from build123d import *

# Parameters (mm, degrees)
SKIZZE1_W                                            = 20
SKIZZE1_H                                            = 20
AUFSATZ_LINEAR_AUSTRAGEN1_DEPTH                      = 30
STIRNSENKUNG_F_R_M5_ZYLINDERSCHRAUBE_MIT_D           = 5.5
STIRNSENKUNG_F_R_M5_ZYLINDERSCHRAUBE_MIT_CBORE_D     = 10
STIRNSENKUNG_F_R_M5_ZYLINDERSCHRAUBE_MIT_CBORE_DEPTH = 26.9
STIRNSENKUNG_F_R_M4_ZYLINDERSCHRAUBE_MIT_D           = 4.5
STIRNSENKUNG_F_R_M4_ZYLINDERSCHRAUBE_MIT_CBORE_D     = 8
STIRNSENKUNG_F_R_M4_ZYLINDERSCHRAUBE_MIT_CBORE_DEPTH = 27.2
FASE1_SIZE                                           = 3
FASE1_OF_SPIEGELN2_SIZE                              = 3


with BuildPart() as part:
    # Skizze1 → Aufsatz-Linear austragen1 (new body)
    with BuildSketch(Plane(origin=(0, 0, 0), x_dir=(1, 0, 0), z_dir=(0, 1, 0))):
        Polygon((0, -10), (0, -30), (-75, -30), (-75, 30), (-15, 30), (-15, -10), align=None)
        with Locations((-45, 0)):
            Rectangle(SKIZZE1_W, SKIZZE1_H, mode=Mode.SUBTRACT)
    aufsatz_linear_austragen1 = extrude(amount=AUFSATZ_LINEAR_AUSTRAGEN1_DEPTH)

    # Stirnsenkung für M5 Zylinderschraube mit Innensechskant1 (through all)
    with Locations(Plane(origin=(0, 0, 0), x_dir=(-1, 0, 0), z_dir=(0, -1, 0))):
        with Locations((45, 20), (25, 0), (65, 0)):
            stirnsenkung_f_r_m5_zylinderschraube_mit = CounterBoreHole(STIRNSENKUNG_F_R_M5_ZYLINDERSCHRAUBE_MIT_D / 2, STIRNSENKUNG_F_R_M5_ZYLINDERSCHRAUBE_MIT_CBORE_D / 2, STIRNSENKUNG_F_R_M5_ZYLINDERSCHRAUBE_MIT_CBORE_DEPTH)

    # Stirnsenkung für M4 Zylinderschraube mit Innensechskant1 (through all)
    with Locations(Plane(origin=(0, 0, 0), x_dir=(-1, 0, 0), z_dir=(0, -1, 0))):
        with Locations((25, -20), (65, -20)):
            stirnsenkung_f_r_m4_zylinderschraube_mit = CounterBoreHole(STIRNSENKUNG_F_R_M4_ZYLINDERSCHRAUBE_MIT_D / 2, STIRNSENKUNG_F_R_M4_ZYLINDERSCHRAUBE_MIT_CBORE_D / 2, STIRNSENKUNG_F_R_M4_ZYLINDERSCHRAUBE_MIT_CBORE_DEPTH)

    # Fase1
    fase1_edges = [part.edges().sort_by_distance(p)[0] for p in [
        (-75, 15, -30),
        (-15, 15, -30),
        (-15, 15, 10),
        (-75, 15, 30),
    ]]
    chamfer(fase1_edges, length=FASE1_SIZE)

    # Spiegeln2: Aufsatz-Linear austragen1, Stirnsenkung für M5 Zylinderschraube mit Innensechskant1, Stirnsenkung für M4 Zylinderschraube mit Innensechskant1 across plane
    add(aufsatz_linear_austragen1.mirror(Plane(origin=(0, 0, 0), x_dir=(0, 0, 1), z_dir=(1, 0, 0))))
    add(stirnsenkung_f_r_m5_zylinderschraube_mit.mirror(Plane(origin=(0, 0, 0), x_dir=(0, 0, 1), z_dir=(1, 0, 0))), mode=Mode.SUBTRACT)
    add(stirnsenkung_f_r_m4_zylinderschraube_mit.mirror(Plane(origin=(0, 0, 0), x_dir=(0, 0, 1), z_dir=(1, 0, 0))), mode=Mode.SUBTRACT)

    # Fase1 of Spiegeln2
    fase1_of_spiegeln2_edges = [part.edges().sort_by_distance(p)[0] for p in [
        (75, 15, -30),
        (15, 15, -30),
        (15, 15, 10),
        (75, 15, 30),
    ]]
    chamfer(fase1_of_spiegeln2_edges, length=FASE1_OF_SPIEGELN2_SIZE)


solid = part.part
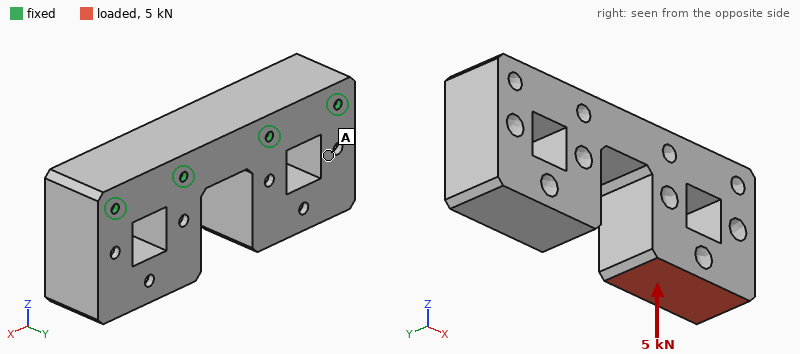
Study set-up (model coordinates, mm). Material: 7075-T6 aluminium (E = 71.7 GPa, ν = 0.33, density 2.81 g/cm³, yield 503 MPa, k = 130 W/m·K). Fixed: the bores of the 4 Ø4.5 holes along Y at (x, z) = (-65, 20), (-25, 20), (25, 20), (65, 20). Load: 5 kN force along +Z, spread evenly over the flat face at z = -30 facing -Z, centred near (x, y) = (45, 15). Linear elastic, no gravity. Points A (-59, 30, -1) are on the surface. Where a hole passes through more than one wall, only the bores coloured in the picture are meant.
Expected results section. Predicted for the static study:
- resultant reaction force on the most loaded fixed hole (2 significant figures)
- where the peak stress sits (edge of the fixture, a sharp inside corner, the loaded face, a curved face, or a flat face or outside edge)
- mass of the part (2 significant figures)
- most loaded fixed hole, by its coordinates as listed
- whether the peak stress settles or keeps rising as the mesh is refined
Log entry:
2.8 kN
edge of the fixture
540 g
(65, 20)
keeps rising
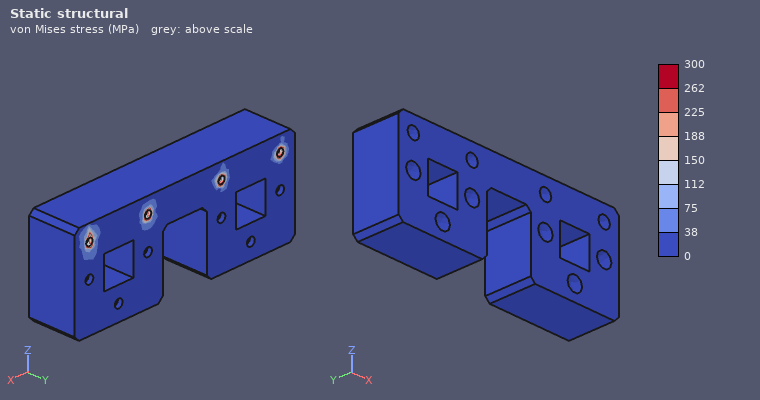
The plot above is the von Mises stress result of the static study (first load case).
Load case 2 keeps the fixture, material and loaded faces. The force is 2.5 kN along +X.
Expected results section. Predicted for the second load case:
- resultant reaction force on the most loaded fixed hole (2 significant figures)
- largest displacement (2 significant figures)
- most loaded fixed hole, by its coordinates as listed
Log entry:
2.4 kN
36 µm
(65, 20)
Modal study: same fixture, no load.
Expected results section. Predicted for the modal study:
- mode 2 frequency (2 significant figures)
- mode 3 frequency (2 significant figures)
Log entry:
2400 Hz
4600 Hz
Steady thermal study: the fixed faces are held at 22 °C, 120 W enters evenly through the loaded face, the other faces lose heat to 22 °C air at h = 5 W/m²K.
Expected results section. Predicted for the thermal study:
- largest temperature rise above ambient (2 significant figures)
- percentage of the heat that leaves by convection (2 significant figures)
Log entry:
67 K
3.6 %
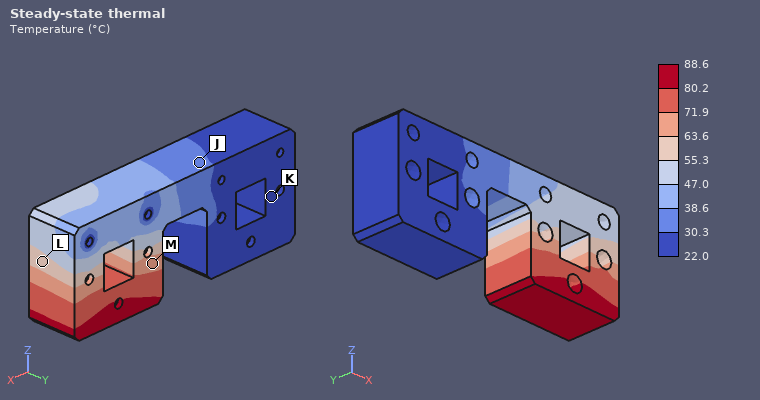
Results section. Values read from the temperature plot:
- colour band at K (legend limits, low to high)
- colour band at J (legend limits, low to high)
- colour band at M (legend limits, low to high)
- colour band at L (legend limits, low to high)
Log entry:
22.0 to 30.3 °C
30.3 to 38.6 °C
63.6 to 71.9 °C
55.3 to 63.6 °C
